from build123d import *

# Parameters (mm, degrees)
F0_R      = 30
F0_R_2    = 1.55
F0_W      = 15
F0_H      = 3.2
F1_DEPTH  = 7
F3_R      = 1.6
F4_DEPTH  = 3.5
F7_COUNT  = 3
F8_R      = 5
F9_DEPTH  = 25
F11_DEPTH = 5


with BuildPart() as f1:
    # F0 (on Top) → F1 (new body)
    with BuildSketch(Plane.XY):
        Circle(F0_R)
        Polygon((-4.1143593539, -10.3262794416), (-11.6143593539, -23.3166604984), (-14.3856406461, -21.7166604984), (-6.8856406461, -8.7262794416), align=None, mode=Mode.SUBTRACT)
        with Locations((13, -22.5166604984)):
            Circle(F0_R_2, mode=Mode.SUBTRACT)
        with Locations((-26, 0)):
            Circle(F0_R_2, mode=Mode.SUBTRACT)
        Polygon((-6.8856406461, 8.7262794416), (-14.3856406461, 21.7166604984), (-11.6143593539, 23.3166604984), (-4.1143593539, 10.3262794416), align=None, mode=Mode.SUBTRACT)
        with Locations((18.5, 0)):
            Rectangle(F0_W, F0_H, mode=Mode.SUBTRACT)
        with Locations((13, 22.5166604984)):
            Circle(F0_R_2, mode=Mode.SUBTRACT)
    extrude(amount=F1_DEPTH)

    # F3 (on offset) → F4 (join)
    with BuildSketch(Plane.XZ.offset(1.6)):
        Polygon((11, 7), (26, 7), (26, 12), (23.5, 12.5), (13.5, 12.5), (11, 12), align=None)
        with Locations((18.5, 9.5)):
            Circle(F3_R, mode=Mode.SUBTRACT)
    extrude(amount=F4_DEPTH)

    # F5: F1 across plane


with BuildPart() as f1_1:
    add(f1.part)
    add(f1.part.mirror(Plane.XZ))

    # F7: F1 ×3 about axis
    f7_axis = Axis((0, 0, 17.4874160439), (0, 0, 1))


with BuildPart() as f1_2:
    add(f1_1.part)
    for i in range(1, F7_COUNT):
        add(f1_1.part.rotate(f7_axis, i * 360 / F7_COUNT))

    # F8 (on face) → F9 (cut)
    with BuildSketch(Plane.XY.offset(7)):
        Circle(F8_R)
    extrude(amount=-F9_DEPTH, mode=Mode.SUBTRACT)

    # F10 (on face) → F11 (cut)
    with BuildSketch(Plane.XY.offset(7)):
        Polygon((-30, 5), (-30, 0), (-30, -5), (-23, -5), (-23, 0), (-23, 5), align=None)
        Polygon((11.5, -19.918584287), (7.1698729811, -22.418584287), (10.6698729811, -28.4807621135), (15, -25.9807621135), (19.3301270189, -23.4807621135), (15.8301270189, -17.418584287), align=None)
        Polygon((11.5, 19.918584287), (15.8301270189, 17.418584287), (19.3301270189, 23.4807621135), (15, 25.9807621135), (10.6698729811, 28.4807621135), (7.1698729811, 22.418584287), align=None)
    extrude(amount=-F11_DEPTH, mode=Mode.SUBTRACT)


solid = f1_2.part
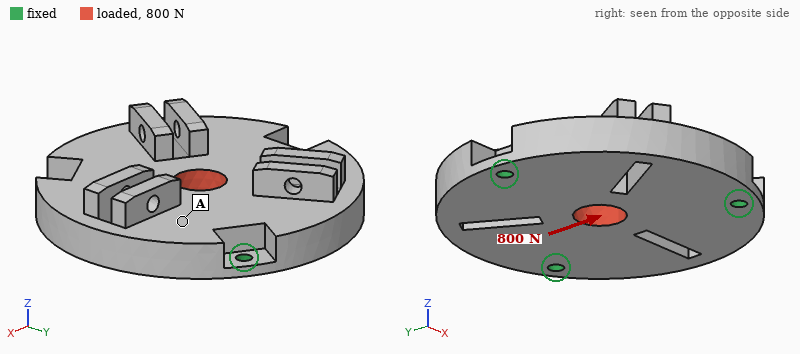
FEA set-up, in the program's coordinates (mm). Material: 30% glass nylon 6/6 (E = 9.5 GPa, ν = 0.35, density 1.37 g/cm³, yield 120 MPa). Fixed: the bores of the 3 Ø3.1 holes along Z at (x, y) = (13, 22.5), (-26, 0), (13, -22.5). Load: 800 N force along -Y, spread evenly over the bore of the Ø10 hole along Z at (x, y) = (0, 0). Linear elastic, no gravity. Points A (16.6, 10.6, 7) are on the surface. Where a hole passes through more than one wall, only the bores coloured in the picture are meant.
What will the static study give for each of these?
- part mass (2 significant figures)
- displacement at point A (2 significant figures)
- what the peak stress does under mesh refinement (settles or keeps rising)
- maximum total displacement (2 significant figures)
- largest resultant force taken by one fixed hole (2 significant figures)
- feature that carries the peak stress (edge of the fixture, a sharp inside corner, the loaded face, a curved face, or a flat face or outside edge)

26 g
9.3 µm
keeps rising
24 µm
300 N
edge of the fixture
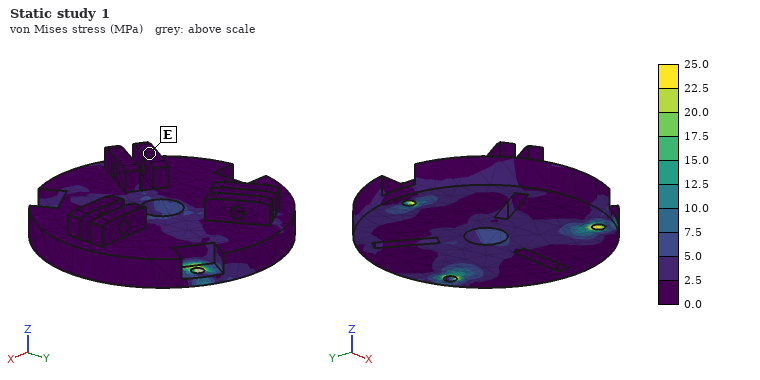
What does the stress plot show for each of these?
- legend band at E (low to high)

0.0 to 2.5 MPa
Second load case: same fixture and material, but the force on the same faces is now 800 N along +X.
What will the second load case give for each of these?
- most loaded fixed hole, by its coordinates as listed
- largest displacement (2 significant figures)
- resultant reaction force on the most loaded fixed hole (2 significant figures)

(-26, 0)
27 µm
320 N
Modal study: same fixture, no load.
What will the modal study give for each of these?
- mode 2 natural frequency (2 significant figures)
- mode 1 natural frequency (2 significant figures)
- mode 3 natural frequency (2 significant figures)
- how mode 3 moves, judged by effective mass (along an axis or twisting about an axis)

3300 Hz
3300 Hz
3800 Hz
along Z
